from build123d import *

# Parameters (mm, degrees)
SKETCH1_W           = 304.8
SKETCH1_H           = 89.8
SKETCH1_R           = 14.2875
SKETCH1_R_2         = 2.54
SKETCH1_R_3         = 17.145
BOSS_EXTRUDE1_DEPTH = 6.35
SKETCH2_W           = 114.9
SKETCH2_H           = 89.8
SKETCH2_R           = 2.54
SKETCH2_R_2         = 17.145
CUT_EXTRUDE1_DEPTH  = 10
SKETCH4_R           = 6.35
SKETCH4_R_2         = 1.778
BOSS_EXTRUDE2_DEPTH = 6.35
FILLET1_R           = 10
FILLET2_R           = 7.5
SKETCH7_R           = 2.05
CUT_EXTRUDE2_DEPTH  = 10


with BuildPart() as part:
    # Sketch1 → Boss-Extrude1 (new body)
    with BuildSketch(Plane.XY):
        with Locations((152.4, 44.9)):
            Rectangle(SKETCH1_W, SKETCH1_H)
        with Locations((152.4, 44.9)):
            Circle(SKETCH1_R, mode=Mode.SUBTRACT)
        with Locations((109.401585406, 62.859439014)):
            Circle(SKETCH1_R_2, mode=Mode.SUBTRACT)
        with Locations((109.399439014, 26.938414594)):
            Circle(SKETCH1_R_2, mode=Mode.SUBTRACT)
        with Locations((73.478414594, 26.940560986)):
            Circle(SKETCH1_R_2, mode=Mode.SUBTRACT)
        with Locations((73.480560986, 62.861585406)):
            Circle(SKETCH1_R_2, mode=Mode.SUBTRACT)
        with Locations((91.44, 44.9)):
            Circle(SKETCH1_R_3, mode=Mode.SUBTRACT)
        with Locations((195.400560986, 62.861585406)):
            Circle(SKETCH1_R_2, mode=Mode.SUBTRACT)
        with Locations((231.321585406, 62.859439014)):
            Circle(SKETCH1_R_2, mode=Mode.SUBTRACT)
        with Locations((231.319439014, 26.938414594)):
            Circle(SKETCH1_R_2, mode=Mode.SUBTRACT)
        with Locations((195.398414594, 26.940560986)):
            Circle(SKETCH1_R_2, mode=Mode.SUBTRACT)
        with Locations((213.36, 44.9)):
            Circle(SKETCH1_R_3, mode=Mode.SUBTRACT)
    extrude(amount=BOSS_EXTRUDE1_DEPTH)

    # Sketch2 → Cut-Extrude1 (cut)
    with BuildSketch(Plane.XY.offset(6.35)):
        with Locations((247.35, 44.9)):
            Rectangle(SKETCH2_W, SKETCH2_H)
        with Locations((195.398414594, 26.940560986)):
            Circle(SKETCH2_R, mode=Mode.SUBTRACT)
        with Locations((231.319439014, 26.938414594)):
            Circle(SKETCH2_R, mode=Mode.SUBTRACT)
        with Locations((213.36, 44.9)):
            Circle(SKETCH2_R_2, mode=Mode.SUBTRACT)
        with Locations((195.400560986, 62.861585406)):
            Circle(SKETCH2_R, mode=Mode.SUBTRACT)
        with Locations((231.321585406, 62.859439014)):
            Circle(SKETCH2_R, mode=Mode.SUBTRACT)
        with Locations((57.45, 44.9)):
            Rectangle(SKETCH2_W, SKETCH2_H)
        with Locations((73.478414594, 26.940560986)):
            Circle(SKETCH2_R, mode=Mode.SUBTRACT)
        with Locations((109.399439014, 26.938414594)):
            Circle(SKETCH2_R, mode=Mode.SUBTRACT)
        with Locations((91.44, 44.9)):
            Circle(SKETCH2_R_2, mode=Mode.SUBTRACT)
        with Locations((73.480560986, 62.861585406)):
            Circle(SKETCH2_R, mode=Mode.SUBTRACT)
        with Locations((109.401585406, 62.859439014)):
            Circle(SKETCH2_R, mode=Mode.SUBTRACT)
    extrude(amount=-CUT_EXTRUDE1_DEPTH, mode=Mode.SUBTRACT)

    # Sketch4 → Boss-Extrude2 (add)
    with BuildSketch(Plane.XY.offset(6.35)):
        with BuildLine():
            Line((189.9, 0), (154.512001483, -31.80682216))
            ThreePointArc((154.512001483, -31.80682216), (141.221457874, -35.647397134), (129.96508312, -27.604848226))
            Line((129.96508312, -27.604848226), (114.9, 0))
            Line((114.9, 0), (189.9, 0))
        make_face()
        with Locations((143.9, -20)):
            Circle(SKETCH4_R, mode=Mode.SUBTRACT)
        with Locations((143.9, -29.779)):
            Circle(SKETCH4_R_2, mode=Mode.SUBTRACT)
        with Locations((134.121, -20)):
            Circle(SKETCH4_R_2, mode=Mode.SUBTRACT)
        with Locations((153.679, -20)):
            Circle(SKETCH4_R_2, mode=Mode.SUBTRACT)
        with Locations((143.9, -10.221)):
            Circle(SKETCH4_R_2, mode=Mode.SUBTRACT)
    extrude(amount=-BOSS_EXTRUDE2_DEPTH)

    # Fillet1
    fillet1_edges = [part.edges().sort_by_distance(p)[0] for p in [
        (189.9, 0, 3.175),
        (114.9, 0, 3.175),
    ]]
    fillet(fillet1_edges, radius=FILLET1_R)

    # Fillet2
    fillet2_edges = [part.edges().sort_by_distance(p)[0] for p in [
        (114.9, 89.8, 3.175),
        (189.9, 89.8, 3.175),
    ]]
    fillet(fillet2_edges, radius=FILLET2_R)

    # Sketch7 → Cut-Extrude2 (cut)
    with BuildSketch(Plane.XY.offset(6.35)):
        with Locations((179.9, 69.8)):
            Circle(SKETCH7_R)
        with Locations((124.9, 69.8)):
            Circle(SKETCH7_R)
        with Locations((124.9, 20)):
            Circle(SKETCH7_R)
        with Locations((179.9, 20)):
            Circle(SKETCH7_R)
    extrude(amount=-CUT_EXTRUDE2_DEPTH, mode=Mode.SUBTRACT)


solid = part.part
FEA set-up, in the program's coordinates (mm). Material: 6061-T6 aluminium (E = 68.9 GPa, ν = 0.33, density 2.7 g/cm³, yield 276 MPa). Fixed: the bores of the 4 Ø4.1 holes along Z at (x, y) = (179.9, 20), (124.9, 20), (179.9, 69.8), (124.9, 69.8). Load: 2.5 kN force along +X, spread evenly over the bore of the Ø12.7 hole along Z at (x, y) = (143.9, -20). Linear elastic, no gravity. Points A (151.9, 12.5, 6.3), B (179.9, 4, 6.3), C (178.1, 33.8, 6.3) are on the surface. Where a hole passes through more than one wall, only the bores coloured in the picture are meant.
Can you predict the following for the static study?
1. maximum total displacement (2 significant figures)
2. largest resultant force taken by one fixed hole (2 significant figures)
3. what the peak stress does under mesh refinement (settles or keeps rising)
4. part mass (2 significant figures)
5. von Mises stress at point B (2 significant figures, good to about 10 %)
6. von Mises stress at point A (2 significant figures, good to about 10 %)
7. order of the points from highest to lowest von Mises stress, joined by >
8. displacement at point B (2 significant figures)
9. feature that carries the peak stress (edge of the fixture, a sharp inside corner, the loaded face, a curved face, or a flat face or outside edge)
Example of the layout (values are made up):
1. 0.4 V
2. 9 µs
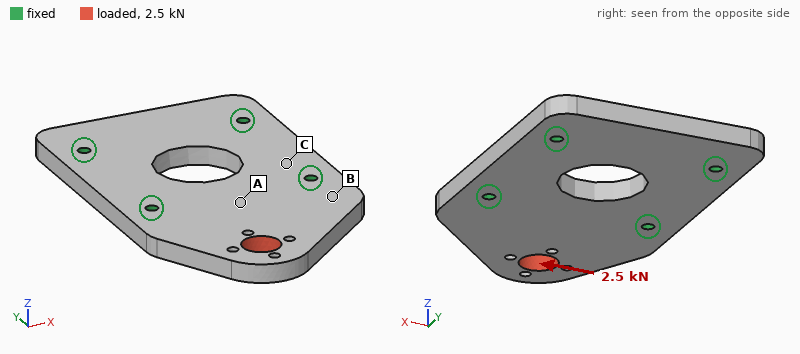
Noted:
1. 24 µm
2. 2.0 kN
3. keeps rising
4. 130 g
5. 12 MPa
6. 8.2 MPa
7. B > A > C
8. 6.5 µm
9. edge of the fixture
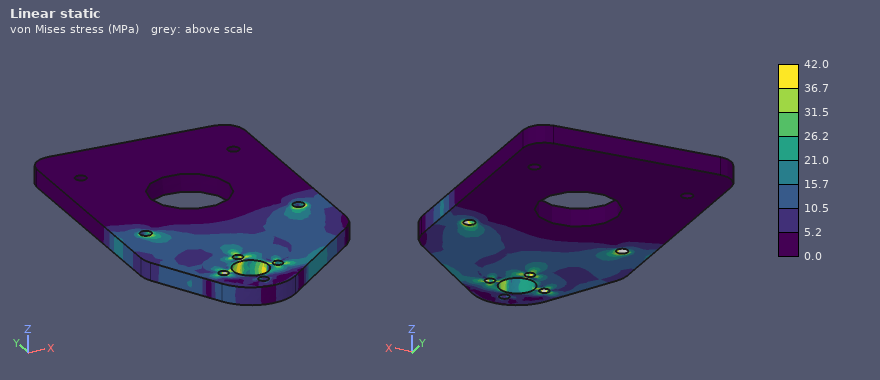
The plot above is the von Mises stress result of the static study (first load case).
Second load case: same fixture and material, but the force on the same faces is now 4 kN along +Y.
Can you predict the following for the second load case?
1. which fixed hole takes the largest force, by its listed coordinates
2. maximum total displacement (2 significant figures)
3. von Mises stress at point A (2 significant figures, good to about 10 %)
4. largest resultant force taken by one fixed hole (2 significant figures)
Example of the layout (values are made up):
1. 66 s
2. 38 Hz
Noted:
1. (124.9, 20)
2. 18 µm
3. 5.6 MPa
4. 2.3 kN
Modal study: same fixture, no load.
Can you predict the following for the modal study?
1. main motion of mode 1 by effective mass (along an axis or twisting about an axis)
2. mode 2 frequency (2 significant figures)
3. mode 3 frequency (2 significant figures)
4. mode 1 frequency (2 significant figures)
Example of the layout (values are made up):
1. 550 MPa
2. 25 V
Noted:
1. along Z
2. 6000 Hz
3. 7400 Hz
4. 2200 Hz
